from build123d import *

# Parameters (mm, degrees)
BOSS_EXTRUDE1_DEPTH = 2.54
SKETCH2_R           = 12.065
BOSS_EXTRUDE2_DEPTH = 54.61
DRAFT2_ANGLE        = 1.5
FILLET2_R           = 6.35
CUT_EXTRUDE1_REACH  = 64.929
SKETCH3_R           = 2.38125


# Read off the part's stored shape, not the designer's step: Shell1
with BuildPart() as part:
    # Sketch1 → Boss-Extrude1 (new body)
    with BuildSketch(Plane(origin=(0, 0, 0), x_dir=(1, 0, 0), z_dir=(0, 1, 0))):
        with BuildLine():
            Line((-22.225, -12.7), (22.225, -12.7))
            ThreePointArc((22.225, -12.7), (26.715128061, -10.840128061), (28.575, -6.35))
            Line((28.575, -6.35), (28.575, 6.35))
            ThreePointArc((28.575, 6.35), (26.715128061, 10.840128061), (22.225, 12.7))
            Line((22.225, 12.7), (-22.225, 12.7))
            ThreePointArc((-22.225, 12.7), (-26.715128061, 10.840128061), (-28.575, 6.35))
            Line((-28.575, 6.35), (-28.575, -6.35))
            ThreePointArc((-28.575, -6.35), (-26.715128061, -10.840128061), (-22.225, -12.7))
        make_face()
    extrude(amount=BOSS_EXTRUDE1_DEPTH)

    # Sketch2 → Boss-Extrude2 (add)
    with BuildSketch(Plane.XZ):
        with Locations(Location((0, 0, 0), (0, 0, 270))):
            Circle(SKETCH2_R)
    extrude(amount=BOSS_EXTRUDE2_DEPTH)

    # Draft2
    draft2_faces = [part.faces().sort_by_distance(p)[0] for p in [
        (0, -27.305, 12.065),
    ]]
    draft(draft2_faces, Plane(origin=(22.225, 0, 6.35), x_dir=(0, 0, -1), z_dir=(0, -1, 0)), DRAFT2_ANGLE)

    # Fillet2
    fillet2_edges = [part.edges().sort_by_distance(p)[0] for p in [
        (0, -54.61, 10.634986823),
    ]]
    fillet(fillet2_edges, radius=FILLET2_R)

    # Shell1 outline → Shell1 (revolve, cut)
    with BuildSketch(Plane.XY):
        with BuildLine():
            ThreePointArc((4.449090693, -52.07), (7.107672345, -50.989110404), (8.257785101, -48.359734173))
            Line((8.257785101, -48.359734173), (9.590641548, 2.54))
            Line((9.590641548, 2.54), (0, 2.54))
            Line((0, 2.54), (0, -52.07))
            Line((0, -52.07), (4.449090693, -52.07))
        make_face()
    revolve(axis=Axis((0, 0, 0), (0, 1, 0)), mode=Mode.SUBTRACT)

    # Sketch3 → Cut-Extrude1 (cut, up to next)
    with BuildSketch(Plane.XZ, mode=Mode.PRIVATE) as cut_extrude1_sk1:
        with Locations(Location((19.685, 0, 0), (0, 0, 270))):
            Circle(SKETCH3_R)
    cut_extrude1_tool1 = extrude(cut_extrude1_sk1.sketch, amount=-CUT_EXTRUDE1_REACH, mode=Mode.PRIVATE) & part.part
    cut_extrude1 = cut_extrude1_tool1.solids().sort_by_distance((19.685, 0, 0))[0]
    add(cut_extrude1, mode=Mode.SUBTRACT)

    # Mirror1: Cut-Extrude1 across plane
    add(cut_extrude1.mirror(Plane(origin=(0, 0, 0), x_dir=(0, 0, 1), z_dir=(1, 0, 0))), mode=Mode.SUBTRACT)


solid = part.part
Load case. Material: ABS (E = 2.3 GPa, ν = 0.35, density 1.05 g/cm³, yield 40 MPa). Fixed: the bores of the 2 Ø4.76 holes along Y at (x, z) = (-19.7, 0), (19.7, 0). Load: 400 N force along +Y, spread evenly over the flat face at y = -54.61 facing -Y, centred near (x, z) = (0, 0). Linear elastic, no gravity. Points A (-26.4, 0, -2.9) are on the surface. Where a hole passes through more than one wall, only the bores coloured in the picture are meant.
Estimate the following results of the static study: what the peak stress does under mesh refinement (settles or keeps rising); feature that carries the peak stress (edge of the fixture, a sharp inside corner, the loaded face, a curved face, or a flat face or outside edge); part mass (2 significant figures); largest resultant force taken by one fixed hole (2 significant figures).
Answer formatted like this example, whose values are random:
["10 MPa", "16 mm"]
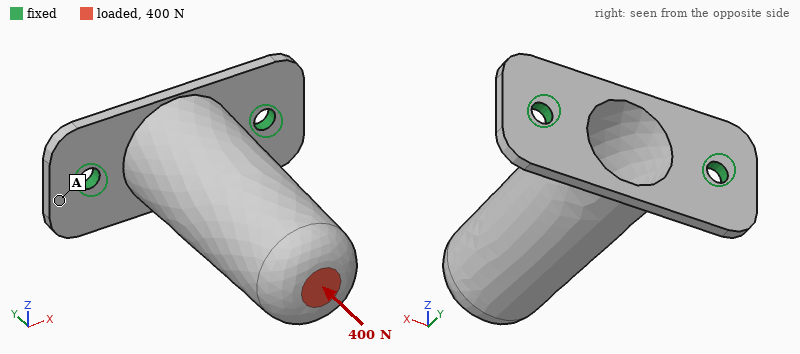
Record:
["keeps rising", "edge of the fixture", "12 g", "210 N"]
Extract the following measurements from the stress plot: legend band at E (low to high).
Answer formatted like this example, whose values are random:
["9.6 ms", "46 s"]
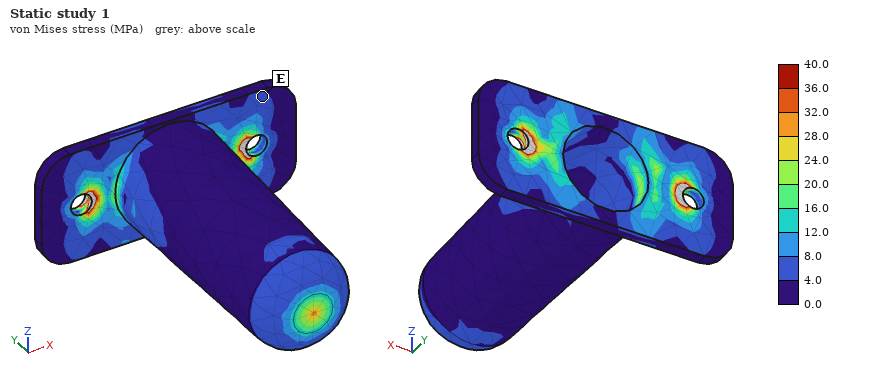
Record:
["4.0 to 8.0 MPa"]
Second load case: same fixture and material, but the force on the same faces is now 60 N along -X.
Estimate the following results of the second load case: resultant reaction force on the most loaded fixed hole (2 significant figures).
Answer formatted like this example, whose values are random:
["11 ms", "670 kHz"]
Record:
["120 N"]
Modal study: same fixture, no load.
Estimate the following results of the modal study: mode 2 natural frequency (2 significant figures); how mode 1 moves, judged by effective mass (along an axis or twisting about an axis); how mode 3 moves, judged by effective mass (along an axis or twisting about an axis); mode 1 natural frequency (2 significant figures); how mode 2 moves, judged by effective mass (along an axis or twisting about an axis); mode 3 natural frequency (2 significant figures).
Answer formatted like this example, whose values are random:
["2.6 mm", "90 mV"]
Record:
["790 Hz", "along Z", "along Y", "280 Hz", "along X", "1700 Hz"]
